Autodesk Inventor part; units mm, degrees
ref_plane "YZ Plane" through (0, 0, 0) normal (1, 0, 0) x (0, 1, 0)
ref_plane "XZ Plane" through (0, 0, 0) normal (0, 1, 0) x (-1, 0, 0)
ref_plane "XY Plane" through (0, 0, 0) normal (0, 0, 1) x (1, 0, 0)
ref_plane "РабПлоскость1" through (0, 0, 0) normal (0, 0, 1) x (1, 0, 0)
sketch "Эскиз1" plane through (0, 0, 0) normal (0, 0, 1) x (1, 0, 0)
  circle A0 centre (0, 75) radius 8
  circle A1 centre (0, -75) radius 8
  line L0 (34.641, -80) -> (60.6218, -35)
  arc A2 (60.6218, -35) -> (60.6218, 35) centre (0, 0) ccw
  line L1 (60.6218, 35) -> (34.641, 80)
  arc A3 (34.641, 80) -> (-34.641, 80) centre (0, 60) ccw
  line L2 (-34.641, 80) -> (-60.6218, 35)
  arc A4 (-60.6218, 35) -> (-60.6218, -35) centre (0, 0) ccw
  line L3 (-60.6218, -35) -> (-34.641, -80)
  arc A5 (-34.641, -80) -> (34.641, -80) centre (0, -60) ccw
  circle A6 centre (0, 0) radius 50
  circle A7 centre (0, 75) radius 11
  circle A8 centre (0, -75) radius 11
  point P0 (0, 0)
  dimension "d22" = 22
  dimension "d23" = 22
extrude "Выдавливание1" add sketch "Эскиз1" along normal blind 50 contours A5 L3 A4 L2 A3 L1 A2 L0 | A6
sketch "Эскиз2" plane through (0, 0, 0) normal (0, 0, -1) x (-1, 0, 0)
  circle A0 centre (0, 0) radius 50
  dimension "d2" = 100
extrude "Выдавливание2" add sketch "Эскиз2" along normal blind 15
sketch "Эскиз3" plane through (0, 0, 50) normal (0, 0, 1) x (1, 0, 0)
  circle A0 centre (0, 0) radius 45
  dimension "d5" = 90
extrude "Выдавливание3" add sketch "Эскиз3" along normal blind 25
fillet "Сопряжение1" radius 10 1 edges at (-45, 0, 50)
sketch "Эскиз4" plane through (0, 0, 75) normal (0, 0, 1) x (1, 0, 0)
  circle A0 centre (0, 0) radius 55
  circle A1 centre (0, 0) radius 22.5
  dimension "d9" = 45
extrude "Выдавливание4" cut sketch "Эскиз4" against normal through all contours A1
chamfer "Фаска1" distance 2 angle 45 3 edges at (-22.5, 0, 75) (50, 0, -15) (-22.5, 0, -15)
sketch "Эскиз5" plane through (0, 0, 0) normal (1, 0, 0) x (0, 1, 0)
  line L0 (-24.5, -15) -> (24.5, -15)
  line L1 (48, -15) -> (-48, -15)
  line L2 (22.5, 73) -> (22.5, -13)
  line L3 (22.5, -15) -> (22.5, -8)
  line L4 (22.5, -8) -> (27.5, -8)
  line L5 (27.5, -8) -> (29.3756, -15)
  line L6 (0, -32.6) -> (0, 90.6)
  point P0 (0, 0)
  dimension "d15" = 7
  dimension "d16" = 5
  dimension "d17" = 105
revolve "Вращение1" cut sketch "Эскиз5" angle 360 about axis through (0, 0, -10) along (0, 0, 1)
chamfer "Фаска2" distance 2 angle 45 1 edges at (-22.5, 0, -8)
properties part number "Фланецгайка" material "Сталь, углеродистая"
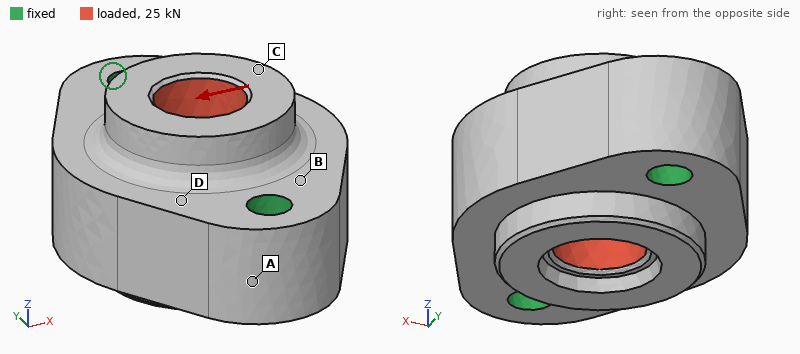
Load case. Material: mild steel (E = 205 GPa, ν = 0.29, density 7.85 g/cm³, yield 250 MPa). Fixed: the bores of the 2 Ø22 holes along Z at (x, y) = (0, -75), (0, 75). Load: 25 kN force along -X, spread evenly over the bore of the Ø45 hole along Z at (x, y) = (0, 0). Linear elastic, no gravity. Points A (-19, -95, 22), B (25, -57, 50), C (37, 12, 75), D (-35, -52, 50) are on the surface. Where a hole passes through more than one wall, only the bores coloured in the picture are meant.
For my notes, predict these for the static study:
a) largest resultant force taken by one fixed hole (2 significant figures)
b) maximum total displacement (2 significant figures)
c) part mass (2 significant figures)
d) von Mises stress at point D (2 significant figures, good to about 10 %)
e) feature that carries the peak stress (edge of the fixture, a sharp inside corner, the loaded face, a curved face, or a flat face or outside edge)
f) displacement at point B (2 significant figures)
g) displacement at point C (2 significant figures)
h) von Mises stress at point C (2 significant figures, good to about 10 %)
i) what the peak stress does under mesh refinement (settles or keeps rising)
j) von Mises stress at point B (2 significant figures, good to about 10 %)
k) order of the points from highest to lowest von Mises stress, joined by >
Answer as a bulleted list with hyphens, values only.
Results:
- 13 kN
- 3.8 µm
- 8.6 kg
- 4.9 MPa
- edge of the fixture
- 1.2 µm
- 3.7 µm
- 2.6 MPa
- keeps rising
- 6.9 MPa
- B > D > C > A
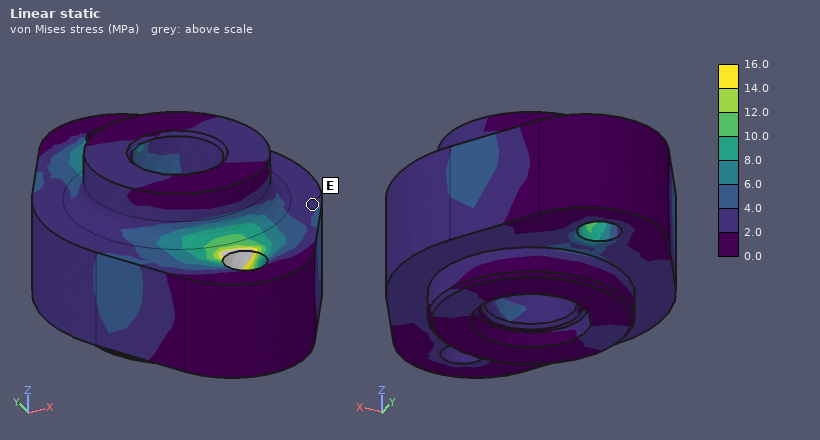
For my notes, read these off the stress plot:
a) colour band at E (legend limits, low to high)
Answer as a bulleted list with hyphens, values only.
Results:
- 2.0 to 4.0 MPa
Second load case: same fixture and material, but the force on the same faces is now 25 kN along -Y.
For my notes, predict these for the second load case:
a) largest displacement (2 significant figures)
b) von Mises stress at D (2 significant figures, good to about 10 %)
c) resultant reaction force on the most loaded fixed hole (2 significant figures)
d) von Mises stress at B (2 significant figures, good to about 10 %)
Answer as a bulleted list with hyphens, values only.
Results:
- 1.6 µm
- 1.8 MPa
- 13 kN
- 2.9 MPa
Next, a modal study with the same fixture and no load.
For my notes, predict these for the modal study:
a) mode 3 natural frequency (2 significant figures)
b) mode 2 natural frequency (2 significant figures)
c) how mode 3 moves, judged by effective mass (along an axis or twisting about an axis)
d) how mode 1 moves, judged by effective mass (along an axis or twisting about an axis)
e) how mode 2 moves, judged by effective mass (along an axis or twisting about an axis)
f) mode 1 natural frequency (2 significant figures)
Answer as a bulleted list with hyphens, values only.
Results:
- 7600 Hz
- 5800 Hz
- along X
- twisting about Y
- along Z
- 4600 Hz
